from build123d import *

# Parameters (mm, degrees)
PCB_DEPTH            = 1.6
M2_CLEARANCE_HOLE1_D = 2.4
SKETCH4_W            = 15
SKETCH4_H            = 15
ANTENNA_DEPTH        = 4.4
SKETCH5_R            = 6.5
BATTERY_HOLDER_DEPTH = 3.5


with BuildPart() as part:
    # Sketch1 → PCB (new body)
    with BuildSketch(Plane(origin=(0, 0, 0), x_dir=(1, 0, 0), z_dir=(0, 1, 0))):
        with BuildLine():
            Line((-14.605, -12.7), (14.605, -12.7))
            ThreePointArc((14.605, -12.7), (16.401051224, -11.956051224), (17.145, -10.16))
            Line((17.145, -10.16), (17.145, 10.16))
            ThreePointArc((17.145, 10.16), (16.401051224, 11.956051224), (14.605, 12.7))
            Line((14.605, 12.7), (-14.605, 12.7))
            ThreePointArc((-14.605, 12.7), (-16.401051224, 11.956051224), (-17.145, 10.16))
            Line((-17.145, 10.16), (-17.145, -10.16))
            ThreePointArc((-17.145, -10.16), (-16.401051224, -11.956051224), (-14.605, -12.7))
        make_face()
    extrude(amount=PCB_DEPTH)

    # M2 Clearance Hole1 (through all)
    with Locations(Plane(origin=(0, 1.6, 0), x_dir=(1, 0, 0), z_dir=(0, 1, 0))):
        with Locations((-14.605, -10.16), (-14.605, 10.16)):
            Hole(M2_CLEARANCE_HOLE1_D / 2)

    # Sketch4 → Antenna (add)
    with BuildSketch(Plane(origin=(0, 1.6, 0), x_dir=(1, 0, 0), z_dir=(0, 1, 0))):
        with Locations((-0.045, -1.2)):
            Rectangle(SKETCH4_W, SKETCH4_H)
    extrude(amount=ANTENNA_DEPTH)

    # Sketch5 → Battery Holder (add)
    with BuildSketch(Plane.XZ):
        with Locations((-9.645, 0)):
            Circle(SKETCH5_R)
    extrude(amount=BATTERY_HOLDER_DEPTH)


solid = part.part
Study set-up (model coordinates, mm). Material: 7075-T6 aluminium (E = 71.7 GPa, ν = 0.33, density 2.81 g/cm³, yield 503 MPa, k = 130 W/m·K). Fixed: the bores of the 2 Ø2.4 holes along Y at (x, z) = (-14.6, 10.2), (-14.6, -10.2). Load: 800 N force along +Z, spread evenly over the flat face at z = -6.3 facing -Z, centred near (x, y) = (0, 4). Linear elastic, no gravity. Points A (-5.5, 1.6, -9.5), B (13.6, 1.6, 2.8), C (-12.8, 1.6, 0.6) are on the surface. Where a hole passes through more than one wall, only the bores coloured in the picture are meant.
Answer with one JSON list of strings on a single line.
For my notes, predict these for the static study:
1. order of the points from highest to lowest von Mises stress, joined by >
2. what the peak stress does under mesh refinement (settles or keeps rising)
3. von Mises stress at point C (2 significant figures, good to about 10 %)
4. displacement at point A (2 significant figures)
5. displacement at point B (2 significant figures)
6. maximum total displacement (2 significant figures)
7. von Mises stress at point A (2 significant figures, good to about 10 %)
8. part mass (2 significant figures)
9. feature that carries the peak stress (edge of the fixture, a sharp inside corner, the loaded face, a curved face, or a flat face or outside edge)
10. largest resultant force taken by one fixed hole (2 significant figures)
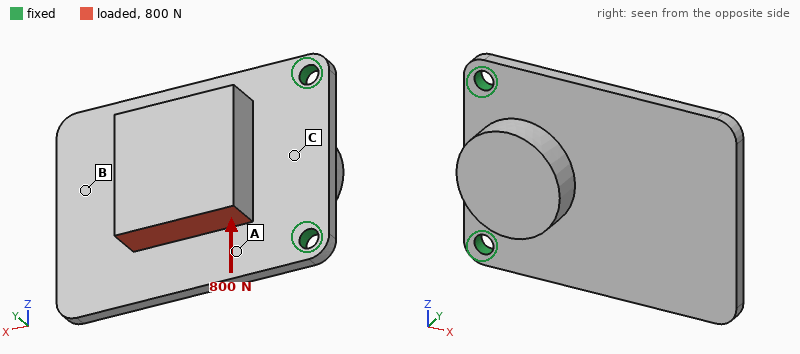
["A > C > B", "keeps rising", "30 MPa", "24 µm", "23 µm", "45 µm", "56 MPa", "7.9 g", "edge of the fixture", "690 N"]
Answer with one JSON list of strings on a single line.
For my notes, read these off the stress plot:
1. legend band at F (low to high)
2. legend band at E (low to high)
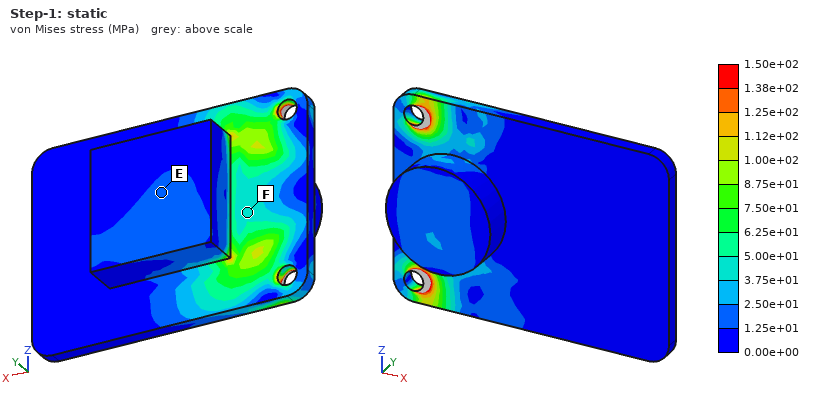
["3.75e+01 to 5.00e+01 MPa", "1.25e+01 to 2.50e+01 MPa"]
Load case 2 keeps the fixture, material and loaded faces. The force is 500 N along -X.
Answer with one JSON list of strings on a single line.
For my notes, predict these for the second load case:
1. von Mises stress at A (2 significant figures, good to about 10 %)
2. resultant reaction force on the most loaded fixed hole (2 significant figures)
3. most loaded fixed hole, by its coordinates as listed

["38 MPa", "410 N", "(-14.6, -10.2)"]
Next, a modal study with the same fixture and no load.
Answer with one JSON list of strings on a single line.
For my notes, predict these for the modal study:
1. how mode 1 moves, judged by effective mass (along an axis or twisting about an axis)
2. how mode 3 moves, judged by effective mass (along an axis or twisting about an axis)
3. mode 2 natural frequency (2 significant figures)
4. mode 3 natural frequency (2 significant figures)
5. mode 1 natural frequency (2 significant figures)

["along Y", "along Y", "8700 Hz", "11 kHz", "1500 Hz"]
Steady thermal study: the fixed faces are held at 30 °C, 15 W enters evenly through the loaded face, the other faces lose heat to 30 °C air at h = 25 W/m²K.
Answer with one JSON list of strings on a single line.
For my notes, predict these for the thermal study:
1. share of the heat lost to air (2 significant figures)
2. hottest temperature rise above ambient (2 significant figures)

["9.2 %", "38 K"]
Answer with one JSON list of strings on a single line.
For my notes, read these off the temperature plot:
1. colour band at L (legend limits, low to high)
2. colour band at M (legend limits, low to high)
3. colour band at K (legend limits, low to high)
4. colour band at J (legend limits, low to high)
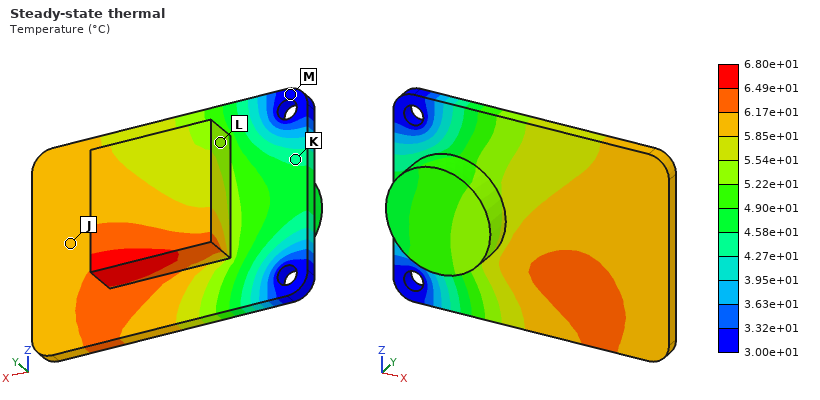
["5.22e+01 to 5.54e+01 °C", "3.00e+01 to 3.32e+01 °C", "4.27e+01 to 4.58e+01 °C", "5.85e+01 to 6.17e+01 °C"]
